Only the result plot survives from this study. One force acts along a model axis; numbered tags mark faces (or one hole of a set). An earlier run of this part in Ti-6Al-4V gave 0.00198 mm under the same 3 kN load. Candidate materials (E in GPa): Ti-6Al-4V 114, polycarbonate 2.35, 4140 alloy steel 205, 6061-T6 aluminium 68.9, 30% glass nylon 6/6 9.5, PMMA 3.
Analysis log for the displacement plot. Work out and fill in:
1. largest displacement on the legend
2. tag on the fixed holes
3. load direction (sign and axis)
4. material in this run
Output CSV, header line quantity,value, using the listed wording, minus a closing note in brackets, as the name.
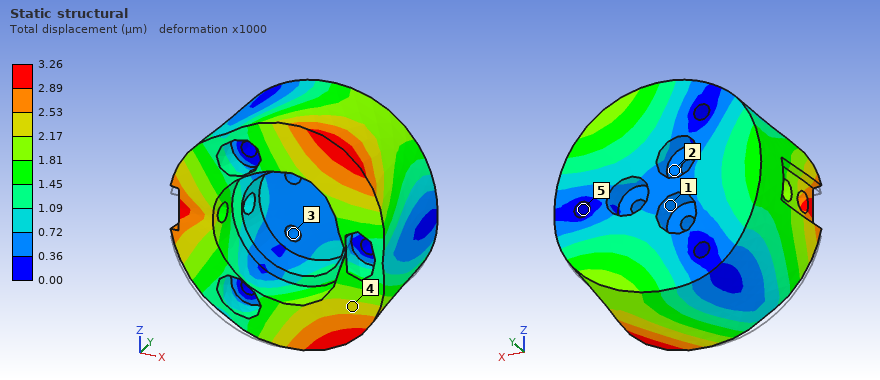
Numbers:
quantity,value
largest displacement on the legend,3.26 µm
tag on the fixed holes,5
load direction,+Y
material in this run,6061-T6 aluminium
